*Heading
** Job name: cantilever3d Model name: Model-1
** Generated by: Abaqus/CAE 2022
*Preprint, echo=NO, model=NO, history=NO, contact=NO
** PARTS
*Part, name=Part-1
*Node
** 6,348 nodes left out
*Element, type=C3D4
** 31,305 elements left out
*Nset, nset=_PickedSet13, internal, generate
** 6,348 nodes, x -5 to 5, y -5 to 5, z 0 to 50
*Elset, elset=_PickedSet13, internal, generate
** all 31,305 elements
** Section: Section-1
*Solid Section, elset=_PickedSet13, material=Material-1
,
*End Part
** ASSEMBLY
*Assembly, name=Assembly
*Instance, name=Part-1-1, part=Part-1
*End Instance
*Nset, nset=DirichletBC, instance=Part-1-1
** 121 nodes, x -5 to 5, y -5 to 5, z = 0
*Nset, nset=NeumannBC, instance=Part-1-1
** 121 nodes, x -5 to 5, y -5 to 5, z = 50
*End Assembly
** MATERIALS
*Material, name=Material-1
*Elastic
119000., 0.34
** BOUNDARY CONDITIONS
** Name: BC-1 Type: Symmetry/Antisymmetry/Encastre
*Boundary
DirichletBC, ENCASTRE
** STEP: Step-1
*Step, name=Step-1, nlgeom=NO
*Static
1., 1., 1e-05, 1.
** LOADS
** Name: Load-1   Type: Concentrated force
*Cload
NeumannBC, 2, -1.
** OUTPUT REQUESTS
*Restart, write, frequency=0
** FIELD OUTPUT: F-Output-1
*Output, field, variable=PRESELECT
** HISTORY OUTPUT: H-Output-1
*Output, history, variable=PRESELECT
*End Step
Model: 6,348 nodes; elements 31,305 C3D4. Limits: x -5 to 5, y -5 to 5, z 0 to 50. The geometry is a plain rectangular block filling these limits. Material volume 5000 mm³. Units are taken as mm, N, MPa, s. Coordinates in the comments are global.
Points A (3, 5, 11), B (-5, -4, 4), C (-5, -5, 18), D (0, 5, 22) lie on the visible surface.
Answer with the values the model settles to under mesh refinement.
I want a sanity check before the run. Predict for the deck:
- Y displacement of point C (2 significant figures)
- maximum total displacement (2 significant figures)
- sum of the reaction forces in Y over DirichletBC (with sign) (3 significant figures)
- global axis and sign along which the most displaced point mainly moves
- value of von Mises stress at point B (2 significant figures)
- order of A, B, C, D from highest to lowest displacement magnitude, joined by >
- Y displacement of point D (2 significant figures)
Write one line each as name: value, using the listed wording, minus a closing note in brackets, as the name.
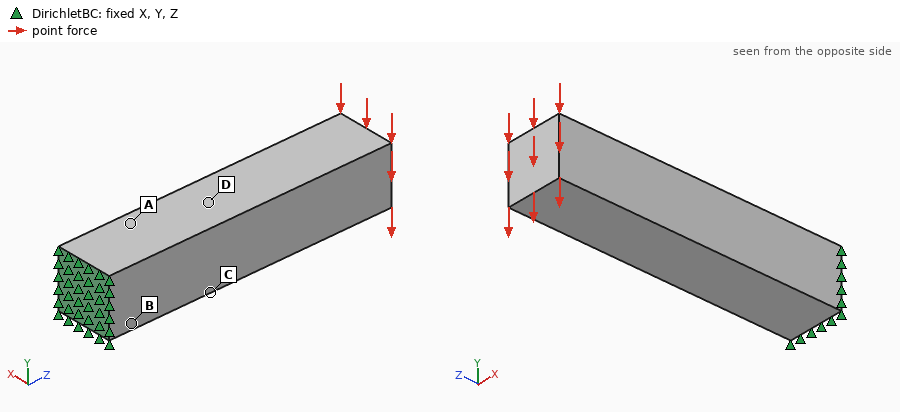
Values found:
Y displacement of point C: -0.0090 mm
maximum total displacement: 0.052 mm
sum of the reaction forces in Y over DirichletBC (with sign): 121 N
global axis and sign along which the most displaced point mainly moves: -Y
value of von Mises stress at point B: 25 MPa
order of A, B, C, D from highest to lowest displacement magnitude, joined by >: D > C > A > B
Y displacement of point D: -0.013 mm
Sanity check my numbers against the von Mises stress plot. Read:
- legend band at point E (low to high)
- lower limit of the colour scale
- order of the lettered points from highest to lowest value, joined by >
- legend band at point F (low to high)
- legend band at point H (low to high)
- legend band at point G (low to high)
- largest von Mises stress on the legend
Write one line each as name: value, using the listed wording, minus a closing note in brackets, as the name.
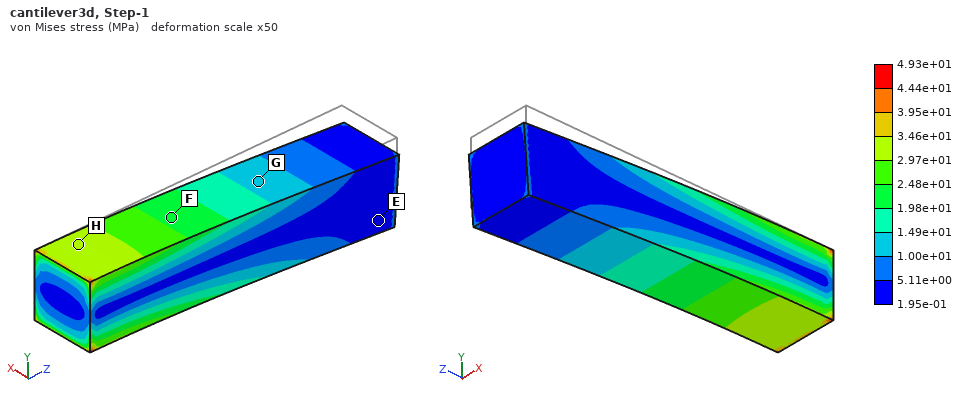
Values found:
legend band at point E: 1.95e-01 to 5.11e+00 MPa
lower limit of the colour scale: 1.95e-01 MPa
order of the lettered points from highest to lowest value, joined by >: H > F > G > E
legend band at point F: 1.98e+01 to 2.48e+01 MPa
legend band at point H: 2.97e+01 to 3.46e+01 MPa
legend band at point G: 1.00e+01 to 1.49e+01 MPa
largest von Mises stress on the legend: 4.93e+01 MPa
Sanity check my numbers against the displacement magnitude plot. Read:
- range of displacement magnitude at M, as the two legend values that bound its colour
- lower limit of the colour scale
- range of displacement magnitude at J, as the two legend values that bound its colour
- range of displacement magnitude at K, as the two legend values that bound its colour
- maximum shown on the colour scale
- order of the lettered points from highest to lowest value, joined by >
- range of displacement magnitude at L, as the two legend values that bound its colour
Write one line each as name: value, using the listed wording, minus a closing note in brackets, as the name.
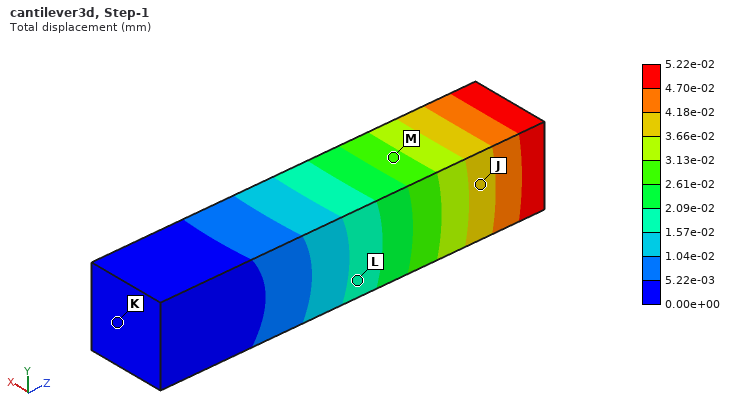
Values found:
range of displacement magnitude at M, as the two legend values that bound its colour: 2.61e-02 to 3.13e-02 mm
lower limit of the colour scale: 0.00e+00 mm
range of displacement magnitude at J, as the two legend values that bound its colour: 3.66e-02 to 4.18e-02 mm
range of displacement magnitude at K, as the two legend values that bound its colour: 0.00e+00 to 5.22e-03 mm
maximum shown on the colour scale: 5.22e-02 mm
order of the lettered points from highest to lowest value, joined by >: J > M > L > K
range of displacement magnitude at L, as the two legend values that bound its colour: 1.57e-02 to 2.09e-02 mm
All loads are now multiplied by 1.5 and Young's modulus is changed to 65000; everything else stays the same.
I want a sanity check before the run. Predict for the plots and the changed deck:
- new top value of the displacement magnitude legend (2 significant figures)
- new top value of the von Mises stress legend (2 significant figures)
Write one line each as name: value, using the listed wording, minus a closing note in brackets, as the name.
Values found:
new top value of the displacement magnitude legend: 0.14 mm
new top value of the von Mises stress legend: 74 MPa
